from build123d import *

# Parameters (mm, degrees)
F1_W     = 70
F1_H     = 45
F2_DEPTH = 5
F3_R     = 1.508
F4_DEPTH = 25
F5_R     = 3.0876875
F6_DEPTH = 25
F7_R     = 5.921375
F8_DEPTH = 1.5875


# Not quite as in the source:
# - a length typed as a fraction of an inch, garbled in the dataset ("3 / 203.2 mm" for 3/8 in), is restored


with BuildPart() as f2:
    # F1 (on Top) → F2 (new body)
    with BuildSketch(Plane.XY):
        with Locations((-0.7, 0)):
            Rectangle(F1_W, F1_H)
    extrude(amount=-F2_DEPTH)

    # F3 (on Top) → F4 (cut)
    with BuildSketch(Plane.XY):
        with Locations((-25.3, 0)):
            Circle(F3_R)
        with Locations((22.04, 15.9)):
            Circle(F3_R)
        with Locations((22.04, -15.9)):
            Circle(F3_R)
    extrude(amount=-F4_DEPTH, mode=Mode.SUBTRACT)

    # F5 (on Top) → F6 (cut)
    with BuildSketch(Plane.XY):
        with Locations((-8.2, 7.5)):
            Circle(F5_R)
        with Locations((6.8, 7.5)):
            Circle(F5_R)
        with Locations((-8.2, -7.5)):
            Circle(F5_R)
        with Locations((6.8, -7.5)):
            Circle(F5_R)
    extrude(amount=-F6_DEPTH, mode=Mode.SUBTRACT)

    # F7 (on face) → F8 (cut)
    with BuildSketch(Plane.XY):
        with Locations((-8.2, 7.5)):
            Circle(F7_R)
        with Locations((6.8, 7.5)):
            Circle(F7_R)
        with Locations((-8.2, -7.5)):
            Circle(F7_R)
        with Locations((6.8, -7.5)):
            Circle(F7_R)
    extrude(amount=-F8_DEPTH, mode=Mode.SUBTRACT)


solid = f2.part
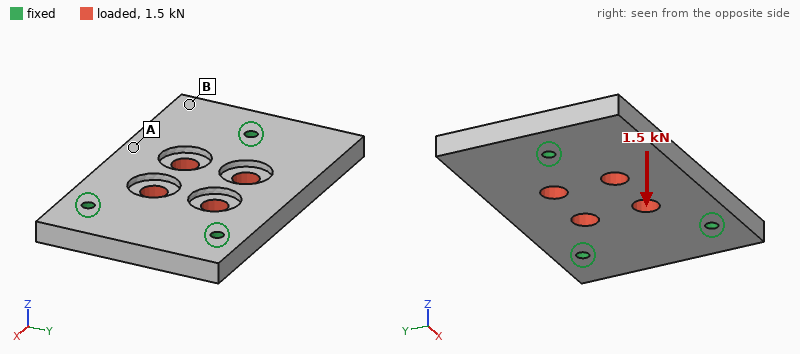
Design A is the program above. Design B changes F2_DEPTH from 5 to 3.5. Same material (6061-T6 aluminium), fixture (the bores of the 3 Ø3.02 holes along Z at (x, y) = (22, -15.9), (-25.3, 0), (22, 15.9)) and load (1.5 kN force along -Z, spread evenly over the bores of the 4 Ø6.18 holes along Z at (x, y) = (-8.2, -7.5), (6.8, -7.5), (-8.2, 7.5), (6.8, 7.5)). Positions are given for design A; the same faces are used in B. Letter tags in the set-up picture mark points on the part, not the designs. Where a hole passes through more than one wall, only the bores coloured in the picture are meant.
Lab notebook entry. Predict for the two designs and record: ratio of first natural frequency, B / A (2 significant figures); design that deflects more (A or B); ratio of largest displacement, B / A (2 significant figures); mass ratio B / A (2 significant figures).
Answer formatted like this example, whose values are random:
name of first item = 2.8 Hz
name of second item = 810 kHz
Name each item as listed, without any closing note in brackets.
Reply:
ratio of first natural frequency, B / A = 0.75
design that deflects more = B
ratio of largest displacement, B / A = 2.7
mass ratio B / A = 0.69
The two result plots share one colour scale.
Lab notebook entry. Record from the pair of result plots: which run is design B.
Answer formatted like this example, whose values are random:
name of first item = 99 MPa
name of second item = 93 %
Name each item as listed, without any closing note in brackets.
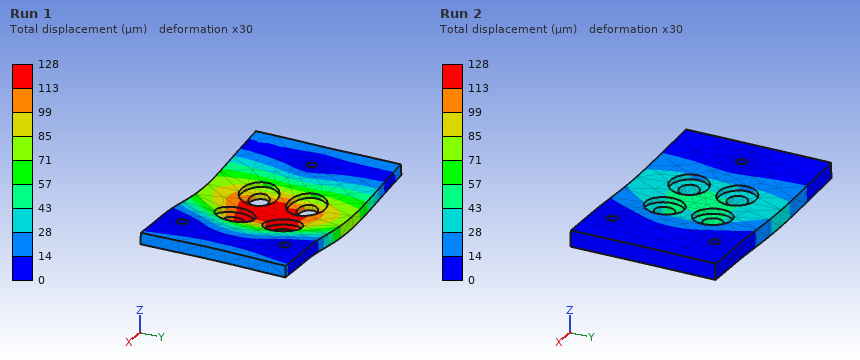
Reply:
which run is design B = Run 1
